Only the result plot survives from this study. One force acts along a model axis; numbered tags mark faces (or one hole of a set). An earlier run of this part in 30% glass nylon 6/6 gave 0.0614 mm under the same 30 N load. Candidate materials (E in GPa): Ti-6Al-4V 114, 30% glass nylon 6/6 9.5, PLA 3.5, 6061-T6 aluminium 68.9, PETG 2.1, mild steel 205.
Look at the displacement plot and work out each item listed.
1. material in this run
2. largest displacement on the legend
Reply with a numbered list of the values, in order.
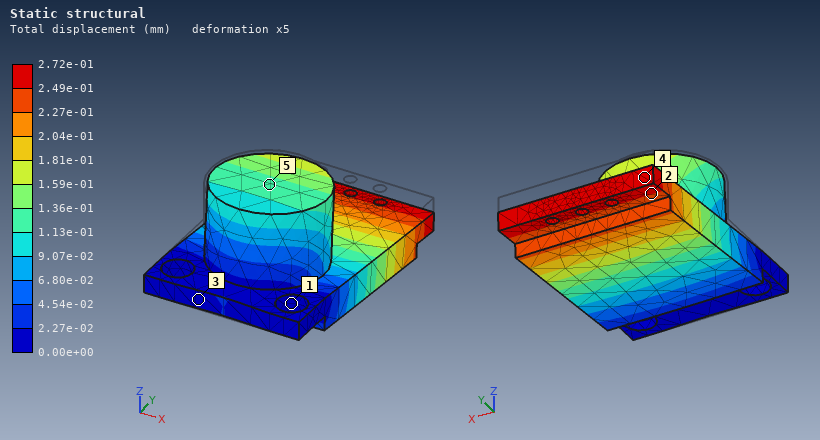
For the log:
1. PETG
2. 2.72e-01 mm
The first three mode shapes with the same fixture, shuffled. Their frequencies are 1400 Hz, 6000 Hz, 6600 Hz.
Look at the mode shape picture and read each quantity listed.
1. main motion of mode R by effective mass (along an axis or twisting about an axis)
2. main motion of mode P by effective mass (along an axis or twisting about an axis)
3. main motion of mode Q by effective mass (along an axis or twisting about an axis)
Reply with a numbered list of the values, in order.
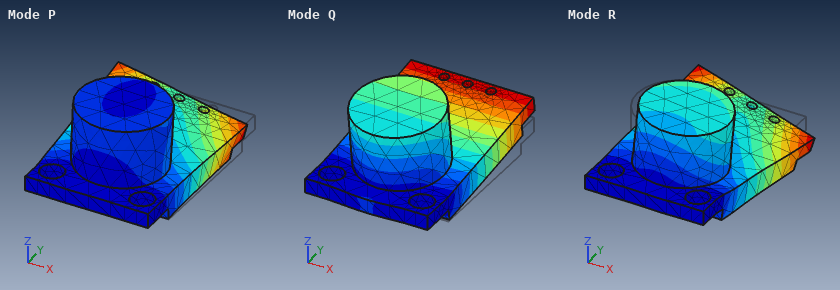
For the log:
1. along X
2. along X
3. along Z
